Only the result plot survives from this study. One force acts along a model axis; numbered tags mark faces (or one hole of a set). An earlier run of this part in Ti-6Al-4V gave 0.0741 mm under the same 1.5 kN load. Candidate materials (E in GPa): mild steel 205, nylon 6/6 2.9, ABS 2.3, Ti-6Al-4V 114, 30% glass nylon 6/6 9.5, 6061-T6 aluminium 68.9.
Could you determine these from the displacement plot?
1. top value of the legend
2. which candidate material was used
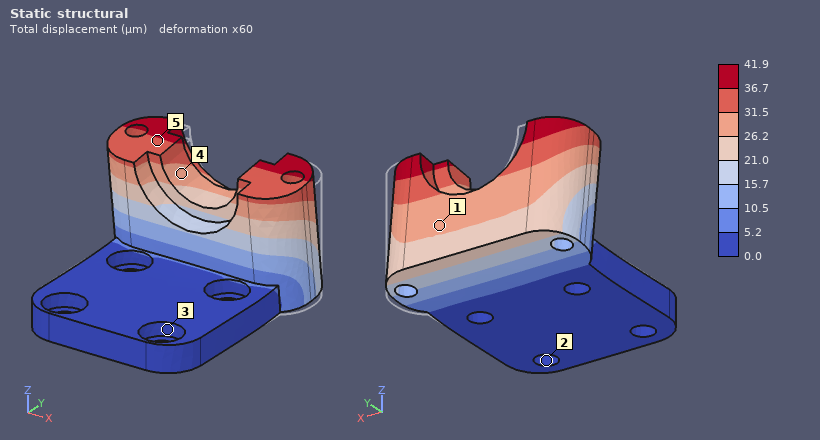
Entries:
41.9 µm
mild steel
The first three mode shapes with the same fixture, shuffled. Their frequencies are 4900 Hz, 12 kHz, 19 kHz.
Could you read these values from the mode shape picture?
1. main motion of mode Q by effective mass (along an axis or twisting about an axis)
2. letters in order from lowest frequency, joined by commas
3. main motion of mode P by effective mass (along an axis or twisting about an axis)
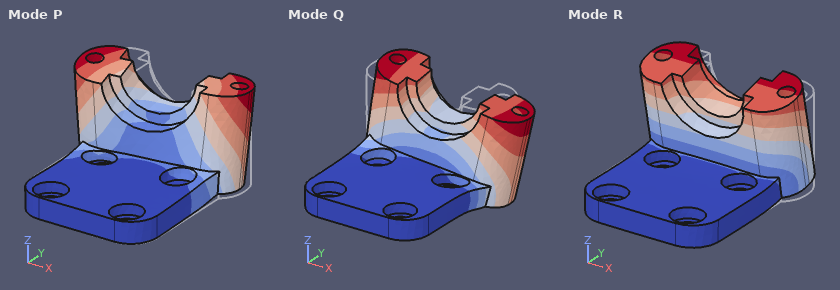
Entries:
along X
R, Q, P
along X
